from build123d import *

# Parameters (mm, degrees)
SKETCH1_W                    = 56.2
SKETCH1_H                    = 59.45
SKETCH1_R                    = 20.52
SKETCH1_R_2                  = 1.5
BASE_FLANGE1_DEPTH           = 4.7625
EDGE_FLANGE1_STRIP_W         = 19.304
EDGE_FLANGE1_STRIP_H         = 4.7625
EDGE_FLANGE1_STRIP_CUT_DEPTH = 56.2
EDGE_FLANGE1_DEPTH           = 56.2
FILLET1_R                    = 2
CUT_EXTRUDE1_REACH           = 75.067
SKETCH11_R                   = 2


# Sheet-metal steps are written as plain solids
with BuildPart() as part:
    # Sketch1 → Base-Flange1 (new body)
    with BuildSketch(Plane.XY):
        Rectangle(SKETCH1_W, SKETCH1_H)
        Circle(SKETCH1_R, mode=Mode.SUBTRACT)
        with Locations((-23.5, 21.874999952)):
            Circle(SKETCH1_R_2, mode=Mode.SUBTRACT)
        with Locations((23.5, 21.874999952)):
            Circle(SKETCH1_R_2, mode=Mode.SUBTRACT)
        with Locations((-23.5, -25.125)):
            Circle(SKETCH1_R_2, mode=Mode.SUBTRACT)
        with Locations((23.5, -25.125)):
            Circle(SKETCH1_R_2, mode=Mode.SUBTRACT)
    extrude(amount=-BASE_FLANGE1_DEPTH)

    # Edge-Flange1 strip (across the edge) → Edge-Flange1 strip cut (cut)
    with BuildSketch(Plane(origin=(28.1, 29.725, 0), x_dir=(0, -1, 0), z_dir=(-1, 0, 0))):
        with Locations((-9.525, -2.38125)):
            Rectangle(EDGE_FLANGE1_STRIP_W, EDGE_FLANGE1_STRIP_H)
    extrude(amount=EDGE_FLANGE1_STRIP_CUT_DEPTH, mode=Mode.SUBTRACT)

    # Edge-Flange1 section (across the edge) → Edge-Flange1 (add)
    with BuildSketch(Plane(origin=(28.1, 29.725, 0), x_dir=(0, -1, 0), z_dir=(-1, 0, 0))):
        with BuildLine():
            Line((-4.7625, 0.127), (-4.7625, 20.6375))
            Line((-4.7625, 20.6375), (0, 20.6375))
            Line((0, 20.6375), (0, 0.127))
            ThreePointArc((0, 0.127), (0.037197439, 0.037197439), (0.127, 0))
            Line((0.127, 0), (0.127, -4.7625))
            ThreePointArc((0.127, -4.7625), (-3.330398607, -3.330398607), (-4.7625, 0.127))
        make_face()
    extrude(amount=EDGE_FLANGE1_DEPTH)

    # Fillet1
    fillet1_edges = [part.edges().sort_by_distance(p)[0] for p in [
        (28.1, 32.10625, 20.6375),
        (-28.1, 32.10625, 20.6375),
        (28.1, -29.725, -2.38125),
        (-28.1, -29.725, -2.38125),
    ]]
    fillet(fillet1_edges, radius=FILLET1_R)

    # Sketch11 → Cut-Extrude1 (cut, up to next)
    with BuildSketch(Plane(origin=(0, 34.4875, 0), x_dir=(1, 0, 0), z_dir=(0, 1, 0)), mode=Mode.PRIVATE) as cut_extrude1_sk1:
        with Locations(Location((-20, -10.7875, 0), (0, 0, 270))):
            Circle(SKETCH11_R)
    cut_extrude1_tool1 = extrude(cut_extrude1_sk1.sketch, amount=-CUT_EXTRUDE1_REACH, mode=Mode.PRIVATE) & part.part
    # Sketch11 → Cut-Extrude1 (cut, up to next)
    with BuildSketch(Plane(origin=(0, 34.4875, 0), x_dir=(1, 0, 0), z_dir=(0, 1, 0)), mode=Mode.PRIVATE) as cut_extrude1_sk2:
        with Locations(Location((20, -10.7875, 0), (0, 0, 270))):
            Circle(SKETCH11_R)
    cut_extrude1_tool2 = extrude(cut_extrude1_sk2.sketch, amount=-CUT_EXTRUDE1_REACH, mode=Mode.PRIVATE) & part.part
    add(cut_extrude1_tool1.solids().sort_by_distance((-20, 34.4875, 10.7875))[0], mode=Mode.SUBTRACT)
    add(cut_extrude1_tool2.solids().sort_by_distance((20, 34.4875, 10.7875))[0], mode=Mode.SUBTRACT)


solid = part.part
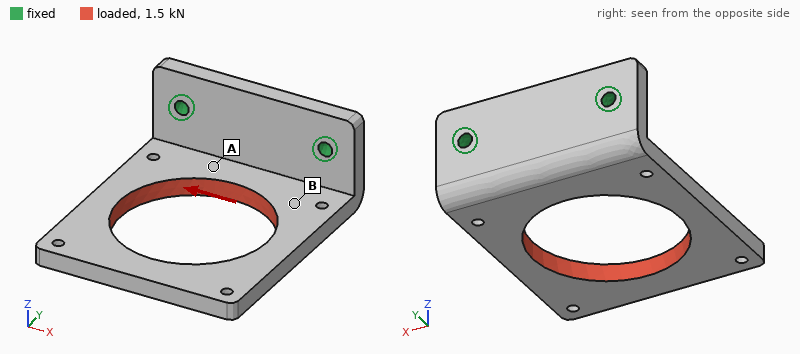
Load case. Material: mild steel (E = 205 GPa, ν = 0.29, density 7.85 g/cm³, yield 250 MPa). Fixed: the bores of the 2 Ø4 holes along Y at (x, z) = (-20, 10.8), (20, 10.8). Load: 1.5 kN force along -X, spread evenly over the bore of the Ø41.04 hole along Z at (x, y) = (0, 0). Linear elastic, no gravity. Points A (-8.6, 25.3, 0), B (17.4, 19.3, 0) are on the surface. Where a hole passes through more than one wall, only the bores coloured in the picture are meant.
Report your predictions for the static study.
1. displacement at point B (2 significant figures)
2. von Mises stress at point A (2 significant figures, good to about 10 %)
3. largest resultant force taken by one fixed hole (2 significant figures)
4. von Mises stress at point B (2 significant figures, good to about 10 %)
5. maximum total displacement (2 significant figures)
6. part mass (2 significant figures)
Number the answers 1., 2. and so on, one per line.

1. 22 µm
2. 56 MPa
3. 1.4 kN
4. 21 MPa
5. 97 µm
6. 120 g
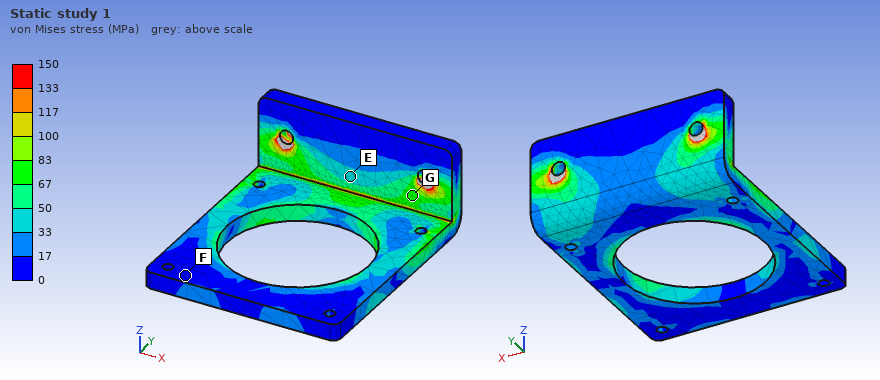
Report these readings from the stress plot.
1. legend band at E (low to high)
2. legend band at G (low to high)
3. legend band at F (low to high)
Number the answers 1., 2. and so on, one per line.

1. 33 to 50 MPa
2. 67 to 83 MPa
3. 0 to 17 MPa
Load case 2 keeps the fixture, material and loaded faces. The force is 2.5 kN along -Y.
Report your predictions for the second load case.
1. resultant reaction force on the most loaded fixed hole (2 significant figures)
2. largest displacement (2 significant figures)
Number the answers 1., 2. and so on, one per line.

1. 1.3 kN
2. 0.17 mm
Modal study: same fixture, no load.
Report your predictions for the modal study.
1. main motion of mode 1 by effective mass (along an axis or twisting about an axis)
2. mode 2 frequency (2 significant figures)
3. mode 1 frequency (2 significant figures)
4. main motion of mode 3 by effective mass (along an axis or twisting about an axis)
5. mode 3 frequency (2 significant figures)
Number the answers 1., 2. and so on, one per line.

1. along Z
2. 1900 Hz
3. 720 Hz
4. along X
5. 2800 Hz
